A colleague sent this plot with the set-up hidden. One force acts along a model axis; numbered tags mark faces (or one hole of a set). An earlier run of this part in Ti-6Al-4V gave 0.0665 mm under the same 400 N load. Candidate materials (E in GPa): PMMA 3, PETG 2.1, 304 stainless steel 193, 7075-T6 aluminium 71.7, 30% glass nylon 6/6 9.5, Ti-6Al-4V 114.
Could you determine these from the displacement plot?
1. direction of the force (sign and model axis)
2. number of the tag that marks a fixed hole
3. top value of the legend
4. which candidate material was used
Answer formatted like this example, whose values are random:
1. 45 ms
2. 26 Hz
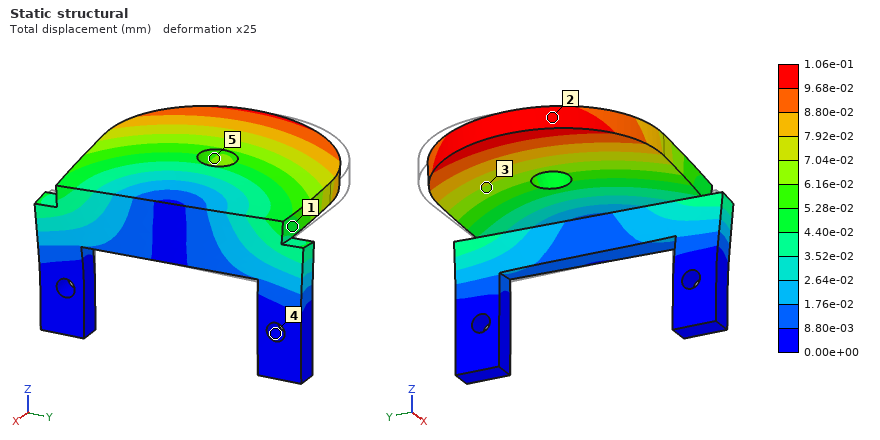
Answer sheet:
1. -Y
2. 4
3. 1.06e-01 mm
4. 7075-T6 aluminium
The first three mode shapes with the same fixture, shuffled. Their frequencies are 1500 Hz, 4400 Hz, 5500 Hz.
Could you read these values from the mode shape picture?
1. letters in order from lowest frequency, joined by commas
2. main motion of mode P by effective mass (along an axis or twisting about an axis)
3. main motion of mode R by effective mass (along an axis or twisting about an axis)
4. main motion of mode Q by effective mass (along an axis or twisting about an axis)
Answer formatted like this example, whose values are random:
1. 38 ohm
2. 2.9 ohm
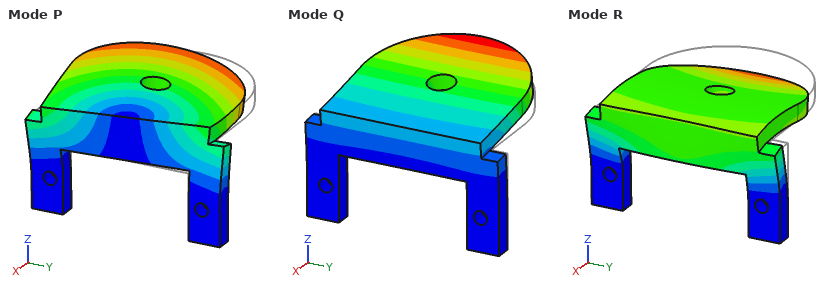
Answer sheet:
1. Q, P, R
2. along Y
3. along X
4. along Z
